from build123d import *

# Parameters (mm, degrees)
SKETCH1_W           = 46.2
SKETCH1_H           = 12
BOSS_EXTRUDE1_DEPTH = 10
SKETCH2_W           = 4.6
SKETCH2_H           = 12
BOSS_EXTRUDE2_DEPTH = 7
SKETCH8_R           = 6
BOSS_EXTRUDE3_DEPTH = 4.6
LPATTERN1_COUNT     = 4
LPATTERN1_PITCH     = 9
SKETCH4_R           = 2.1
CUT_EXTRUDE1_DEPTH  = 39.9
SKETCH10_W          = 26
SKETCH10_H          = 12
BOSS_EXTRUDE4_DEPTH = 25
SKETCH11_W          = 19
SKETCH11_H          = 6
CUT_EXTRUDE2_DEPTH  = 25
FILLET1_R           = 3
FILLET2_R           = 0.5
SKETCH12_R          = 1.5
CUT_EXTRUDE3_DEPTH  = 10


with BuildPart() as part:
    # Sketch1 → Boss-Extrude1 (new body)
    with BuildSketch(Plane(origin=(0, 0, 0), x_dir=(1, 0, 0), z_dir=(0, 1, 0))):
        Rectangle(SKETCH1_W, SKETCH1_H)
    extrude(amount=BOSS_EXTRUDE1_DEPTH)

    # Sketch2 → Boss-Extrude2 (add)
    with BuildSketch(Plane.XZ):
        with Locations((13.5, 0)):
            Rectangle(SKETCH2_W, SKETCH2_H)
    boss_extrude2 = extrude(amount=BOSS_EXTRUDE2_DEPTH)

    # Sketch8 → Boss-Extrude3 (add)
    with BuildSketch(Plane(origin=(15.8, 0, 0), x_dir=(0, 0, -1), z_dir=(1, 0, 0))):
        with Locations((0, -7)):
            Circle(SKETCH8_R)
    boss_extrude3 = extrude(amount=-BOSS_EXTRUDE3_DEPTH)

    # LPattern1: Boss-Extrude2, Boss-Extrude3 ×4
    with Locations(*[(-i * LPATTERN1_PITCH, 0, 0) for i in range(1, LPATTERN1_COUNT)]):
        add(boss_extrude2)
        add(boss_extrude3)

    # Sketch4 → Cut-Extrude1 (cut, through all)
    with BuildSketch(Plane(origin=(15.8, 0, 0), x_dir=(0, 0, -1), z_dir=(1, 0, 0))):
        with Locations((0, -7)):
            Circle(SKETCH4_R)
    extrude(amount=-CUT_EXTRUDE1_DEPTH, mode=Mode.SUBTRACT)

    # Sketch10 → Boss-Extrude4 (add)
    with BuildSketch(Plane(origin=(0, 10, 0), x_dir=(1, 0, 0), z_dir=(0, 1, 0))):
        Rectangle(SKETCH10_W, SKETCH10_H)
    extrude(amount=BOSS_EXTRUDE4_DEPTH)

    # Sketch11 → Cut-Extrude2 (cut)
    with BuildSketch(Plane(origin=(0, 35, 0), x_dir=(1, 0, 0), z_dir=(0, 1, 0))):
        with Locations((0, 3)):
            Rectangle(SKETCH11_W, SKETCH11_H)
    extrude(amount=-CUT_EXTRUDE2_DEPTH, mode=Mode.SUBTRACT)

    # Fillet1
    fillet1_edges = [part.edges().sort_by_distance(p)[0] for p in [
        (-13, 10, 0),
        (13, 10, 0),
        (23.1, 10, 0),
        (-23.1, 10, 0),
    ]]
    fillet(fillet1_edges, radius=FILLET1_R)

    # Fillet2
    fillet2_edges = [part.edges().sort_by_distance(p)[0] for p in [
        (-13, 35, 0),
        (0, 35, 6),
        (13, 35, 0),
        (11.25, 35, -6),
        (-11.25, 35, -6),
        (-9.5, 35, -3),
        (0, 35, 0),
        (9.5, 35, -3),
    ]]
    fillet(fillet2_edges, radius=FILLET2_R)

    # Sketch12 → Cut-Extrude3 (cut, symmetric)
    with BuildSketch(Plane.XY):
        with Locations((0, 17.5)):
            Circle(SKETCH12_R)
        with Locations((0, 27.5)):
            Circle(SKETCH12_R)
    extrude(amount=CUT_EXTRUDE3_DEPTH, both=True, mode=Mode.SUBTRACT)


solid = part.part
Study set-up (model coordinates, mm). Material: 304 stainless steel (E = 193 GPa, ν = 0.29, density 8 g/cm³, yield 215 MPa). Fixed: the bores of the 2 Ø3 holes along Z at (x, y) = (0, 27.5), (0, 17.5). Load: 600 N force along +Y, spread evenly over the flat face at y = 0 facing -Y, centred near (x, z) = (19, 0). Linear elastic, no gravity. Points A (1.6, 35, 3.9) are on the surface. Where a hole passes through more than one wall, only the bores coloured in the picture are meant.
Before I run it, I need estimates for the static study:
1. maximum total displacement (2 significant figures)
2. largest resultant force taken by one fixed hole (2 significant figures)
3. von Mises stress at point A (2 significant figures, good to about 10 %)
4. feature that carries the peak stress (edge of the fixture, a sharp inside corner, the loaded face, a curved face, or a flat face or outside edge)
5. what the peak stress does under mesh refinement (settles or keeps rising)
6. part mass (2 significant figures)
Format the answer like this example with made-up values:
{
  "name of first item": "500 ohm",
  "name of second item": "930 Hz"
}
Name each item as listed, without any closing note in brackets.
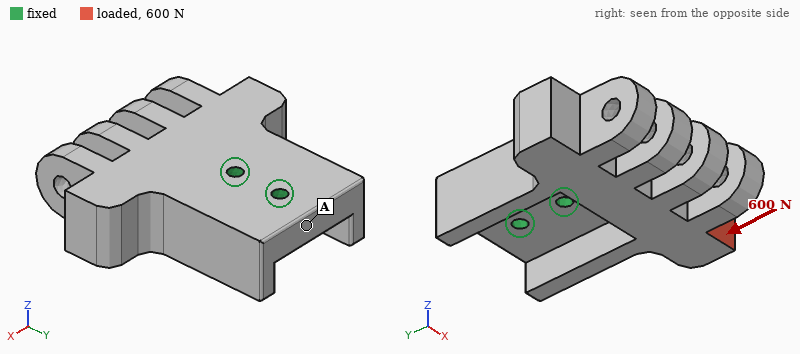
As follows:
{
  "maximum total displacement": "10 µm",
  "largest resultant force taken by one fixed hole": "970 N",
  "von Mises stress at point A": "5.6 MPa",
  "feature that carries the peak stress": "edge of the fixture",
  "what the peak stress does under mesh refinement": "keeps rising",
  "part mass": "100 g"
}
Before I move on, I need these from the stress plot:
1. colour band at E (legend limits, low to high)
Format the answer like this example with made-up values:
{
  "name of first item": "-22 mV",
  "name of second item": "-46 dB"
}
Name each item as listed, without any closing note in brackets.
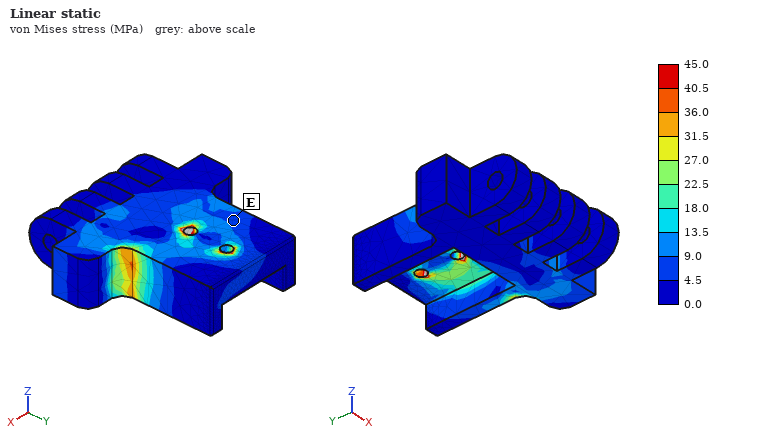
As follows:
{
  "colour band at E": "4.5 to 9.0 MPa"
}
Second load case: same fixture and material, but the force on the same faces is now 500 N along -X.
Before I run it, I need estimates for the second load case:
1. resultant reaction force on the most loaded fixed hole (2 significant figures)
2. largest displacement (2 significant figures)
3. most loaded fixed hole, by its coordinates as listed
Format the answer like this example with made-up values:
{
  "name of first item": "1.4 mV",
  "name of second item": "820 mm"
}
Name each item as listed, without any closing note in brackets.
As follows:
{
  "resultant reaction force on the most loaded fixed hole": "1.2 kN",
  "largest displacement": "7.2 µm",
  "most loaded fixed hole, by its coordinates as listed": "(0, 17.5)"
}
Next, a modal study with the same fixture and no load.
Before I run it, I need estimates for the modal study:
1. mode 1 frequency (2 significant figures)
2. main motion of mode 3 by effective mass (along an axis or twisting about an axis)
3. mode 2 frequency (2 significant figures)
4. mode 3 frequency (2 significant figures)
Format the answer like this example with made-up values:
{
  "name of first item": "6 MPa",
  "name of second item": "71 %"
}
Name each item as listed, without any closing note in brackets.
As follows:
{
  "mode 1 frequency": "5100 Hz",
  "main motion of mode 3 by effective mass": "along X",
  "mode 2 frequency": "5200 Hz",
  "mode 3 frequency": "7000 Hz"
}
